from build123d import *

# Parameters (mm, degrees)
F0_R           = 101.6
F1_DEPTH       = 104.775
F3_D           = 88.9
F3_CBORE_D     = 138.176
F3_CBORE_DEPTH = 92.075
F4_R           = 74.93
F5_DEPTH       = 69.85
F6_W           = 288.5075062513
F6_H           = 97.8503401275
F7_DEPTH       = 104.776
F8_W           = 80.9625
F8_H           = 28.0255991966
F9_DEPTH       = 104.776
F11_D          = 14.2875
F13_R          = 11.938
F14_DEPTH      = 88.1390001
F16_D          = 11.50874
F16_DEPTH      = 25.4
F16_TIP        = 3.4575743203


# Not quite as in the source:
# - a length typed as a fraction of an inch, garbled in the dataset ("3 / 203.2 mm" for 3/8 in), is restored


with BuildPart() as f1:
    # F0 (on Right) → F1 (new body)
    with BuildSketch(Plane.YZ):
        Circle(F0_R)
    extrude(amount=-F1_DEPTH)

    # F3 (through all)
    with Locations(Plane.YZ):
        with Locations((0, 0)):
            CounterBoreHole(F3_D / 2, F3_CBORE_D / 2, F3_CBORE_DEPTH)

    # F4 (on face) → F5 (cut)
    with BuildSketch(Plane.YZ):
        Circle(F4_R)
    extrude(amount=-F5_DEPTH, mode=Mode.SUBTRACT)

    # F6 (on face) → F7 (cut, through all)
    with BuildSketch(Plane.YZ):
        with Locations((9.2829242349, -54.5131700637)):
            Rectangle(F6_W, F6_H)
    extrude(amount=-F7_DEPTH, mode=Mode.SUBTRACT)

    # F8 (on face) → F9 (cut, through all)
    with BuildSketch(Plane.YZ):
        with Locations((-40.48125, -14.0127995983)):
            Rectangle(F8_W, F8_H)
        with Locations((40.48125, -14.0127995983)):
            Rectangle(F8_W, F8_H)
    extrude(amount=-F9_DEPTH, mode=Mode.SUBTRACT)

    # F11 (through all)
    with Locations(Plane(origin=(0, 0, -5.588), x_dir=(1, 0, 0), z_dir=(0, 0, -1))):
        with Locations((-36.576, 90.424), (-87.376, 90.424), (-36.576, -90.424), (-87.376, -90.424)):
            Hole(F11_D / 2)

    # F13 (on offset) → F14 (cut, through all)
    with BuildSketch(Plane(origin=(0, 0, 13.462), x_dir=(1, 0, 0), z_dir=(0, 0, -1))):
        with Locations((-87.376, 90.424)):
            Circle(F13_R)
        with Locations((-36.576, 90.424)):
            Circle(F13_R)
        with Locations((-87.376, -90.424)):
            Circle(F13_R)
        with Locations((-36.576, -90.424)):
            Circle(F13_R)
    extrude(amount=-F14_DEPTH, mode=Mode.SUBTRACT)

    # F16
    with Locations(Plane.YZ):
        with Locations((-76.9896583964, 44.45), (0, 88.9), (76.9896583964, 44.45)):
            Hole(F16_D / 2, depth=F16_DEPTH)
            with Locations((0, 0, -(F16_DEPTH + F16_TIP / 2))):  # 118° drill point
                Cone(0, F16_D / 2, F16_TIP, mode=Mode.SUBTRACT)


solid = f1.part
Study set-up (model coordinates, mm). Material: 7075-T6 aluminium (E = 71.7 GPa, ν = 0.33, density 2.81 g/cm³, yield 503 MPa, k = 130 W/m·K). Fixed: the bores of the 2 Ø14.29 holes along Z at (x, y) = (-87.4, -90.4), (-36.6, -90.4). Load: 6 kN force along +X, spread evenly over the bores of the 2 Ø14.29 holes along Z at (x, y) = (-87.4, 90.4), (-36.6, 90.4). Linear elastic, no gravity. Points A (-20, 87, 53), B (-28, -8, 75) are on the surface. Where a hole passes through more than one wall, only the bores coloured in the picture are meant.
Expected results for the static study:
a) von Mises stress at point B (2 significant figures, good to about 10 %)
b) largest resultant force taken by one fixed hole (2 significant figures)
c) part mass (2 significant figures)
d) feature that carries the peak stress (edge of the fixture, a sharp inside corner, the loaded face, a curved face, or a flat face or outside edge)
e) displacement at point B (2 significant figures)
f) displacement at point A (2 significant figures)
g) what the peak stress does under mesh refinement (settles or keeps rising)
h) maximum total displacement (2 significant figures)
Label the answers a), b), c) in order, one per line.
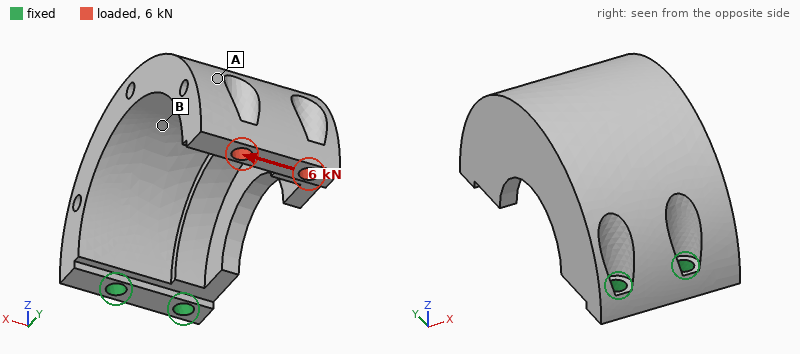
a) 48 MPa
b) 15 kN
c) 2.3 kg
d) edge of the fixture
e) 0.30 mm
f) 0.85 mm
g) keeps rising
h) 1.3 mm
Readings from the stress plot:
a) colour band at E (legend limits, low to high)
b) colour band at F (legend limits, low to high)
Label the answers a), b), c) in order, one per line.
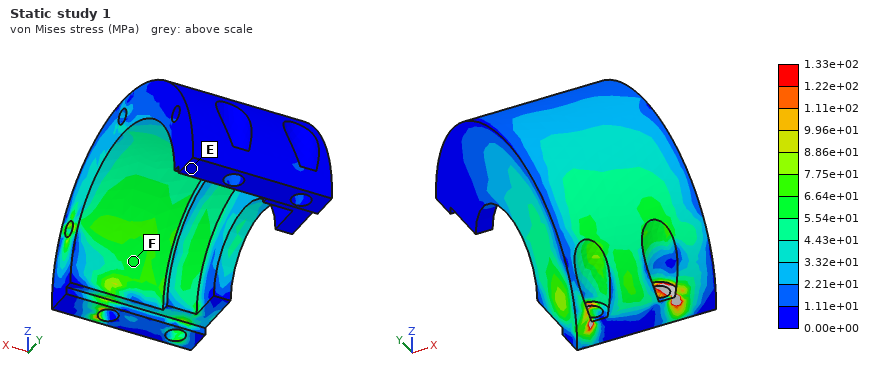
a) 0.00e+00 to 1.11e+01 MPa
b) 5.54e+01 to 6.64e+01 MPa
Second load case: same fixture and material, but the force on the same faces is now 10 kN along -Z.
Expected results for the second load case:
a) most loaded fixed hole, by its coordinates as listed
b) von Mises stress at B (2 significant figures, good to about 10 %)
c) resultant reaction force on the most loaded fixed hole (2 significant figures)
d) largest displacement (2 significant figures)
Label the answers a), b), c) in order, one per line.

a) (-87.4, -90.4)
b) 44 MPa
c) 7.4 kN
d) 2.7 mm
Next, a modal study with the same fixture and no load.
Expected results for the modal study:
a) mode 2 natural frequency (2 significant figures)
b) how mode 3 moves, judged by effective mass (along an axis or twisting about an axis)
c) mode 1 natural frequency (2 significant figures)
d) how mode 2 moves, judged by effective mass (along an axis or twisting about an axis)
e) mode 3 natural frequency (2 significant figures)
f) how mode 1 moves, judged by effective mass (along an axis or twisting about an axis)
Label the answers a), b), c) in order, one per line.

a) 500 Hz
b) along Y
c) 350 Hz
d) along X
e) 1300 Hz
f) along Z
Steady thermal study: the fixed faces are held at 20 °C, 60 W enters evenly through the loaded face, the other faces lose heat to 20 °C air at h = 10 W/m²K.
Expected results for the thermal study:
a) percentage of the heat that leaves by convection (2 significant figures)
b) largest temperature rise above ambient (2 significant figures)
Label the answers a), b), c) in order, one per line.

a) 28 %
b) 38 K
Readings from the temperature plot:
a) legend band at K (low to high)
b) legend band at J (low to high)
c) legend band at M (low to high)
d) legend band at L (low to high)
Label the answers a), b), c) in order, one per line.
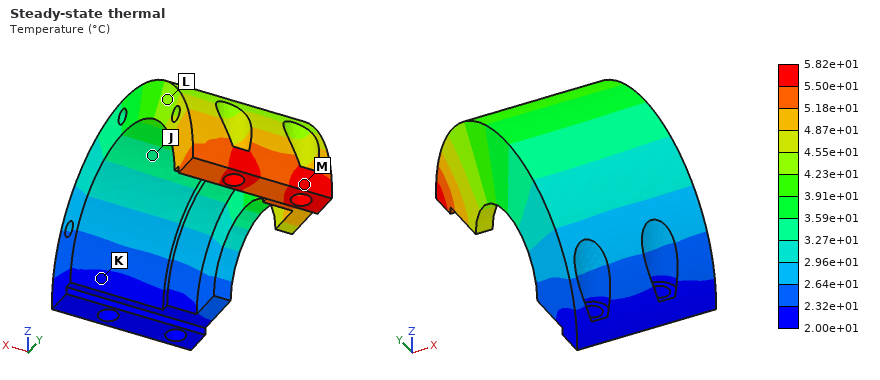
a) 2.00e+01 to 2.32e+01 °C
b) 3.27e+01 to 3.59e+01 °C
c) 5.50e+01 to 5.82e+01 °C
d) 4.23e+01 to 4.55e+01 °C
